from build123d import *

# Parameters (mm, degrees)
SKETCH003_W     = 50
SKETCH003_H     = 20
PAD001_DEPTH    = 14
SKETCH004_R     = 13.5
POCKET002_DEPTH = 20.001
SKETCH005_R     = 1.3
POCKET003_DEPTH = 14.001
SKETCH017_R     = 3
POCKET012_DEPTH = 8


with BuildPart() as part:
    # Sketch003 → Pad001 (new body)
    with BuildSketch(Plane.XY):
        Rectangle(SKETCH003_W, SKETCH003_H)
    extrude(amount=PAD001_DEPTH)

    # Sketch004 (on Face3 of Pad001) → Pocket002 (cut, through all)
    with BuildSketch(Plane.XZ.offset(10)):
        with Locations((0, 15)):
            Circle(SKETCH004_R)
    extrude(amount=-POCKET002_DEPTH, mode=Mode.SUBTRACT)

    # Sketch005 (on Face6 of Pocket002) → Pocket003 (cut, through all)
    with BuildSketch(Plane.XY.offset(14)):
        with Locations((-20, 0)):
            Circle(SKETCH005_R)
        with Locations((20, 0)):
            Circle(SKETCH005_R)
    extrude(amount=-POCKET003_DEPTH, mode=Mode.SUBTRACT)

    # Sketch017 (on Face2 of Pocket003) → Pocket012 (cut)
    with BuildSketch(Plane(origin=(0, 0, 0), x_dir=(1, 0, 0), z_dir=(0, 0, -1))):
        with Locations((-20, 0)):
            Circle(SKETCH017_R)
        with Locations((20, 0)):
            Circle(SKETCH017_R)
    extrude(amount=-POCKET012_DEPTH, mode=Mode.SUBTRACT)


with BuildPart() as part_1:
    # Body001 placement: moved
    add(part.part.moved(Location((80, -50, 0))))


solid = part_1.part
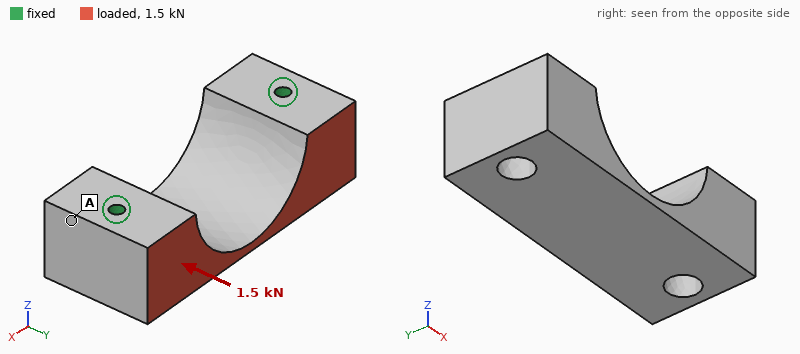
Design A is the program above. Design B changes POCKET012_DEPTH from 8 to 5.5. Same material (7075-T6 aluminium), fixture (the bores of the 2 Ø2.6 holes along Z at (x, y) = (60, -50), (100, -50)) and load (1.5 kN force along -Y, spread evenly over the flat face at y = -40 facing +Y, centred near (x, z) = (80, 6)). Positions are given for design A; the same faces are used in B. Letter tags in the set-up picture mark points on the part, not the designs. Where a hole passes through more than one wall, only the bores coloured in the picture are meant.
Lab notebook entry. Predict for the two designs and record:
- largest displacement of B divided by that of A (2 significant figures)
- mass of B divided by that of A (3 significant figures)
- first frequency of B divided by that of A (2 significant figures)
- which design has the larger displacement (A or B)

0.55
1.01
1.4
A
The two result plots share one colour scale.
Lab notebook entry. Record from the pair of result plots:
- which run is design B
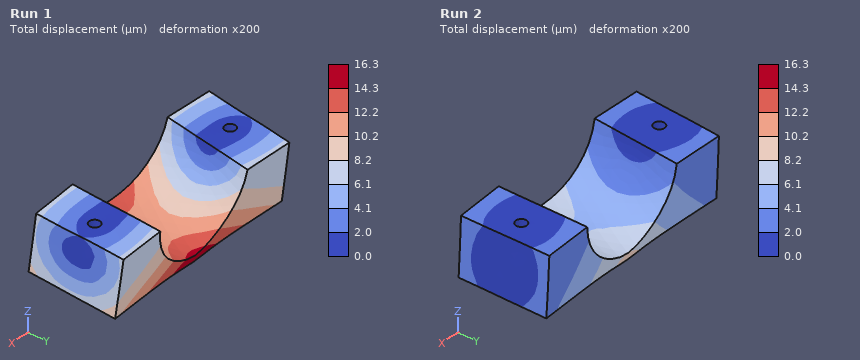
Run 2
